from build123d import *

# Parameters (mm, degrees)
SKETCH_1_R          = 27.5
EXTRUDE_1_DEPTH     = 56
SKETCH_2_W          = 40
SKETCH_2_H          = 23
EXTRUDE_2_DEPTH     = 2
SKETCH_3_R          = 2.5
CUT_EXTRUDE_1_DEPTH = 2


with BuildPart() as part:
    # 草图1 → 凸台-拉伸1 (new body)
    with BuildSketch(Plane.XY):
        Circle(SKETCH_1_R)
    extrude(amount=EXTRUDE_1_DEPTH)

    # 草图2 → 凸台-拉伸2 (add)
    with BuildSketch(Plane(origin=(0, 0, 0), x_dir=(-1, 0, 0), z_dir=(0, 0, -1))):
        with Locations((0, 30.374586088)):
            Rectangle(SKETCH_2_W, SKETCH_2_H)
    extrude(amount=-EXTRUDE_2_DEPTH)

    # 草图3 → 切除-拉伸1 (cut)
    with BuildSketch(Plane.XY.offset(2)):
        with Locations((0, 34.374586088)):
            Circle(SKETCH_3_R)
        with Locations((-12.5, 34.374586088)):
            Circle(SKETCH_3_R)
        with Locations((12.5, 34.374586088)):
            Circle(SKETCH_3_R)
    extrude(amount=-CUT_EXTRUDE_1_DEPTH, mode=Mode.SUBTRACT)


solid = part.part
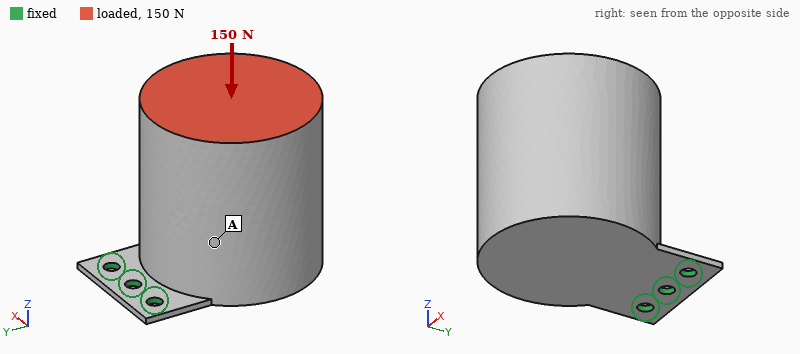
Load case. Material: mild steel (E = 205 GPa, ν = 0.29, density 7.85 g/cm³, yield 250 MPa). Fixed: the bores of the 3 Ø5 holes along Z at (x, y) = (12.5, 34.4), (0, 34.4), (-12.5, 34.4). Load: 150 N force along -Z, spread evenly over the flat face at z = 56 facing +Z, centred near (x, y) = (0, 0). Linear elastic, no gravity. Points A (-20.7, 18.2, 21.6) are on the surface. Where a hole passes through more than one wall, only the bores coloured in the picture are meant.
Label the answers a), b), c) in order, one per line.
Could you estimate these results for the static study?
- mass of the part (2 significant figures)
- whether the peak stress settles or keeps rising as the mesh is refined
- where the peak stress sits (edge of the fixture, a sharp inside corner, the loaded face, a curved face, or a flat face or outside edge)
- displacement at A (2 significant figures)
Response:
a) 1.1 kg
b) keeps rising
c) edge of the fixture
d) 0.13 mm
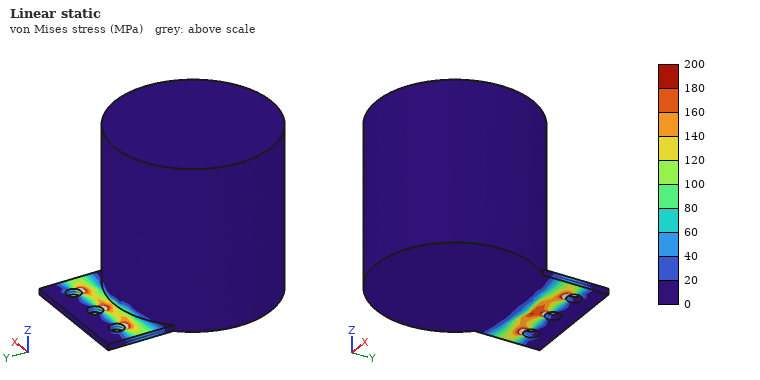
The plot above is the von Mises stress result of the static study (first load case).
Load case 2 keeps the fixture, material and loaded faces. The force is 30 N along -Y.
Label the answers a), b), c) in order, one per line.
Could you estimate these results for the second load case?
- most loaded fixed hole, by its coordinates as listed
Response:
a) (0, 34.4)
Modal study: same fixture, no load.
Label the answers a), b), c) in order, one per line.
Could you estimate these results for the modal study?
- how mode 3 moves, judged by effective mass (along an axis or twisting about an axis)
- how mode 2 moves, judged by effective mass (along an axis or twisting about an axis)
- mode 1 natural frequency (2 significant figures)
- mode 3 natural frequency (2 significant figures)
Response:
a) along X
b) along X
c) 96 Hz
d) 2000 Hz
